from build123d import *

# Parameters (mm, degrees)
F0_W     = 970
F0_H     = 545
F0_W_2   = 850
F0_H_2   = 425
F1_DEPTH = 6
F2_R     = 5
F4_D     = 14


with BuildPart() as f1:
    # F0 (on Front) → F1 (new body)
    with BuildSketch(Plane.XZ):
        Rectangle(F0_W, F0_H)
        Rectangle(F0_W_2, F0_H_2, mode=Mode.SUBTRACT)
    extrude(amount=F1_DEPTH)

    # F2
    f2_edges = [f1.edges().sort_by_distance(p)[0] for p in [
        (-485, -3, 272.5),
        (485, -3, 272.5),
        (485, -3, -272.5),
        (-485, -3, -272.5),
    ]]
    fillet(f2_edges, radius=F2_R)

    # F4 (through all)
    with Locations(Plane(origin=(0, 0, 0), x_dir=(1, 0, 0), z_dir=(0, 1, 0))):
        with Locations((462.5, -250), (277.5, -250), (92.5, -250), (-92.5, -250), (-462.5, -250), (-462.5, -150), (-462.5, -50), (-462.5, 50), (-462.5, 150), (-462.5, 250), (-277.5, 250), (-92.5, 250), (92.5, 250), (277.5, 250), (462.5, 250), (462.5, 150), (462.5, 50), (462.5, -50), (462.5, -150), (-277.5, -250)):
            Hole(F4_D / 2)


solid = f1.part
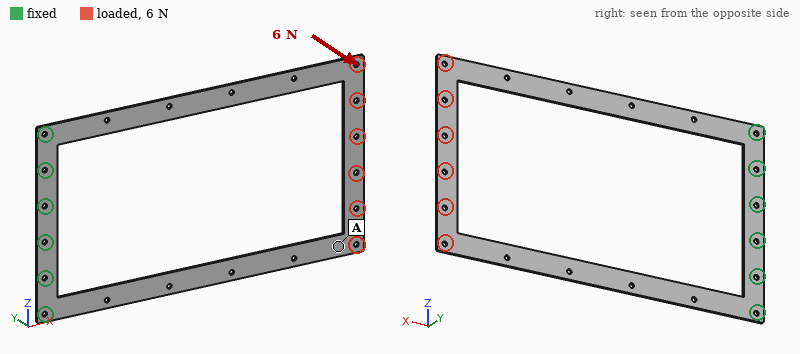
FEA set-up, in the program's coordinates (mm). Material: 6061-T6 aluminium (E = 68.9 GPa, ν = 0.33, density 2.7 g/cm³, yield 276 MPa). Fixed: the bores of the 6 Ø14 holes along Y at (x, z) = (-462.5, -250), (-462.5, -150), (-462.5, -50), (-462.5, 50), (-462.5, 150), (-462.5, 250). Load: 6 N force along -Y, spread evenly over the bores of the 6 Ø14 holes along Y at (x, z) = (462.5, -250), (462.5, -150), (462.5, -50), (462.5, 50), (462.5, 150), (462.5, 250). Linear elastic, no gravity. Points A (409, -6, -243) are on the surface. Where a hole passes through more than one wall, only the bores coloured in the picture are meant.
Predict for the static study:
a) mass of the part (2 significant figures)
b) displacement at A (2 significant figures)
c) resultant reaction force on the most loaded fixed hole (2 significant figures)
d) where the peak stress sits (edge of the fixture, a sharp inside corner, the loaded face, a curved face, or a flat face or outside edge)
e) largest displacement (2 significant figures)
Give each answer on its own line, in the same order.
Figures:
2.7 kg
9.6 mm
6.1 N
a curved face
11 mm
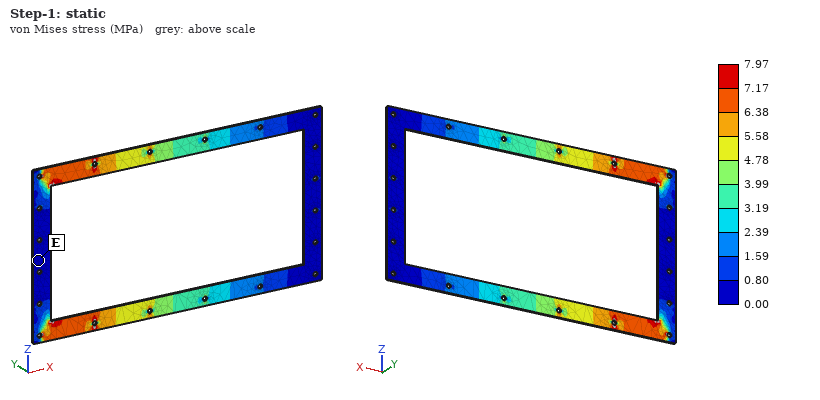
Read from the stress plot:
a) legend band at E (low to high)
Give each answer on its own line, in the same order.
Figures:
0.00 to 0.80 MPa
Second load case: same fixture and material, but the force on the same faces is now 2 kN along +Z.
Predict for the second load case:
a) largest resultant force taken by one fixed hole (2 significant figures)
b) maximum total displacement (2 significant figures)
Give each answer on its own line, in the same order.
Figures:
6.5 kN
11 mm
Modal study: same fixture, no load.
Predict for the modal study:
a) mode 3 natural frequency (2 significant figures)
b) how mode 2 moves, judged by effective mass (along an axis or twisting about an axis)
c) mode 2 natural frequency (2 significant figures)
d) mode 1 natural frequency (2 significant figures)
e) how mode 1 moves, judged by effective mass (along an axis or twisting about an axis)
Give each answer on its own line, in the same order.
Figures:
29 Hz
twisting about X
13 Hz
4.1 Hz
along Y
